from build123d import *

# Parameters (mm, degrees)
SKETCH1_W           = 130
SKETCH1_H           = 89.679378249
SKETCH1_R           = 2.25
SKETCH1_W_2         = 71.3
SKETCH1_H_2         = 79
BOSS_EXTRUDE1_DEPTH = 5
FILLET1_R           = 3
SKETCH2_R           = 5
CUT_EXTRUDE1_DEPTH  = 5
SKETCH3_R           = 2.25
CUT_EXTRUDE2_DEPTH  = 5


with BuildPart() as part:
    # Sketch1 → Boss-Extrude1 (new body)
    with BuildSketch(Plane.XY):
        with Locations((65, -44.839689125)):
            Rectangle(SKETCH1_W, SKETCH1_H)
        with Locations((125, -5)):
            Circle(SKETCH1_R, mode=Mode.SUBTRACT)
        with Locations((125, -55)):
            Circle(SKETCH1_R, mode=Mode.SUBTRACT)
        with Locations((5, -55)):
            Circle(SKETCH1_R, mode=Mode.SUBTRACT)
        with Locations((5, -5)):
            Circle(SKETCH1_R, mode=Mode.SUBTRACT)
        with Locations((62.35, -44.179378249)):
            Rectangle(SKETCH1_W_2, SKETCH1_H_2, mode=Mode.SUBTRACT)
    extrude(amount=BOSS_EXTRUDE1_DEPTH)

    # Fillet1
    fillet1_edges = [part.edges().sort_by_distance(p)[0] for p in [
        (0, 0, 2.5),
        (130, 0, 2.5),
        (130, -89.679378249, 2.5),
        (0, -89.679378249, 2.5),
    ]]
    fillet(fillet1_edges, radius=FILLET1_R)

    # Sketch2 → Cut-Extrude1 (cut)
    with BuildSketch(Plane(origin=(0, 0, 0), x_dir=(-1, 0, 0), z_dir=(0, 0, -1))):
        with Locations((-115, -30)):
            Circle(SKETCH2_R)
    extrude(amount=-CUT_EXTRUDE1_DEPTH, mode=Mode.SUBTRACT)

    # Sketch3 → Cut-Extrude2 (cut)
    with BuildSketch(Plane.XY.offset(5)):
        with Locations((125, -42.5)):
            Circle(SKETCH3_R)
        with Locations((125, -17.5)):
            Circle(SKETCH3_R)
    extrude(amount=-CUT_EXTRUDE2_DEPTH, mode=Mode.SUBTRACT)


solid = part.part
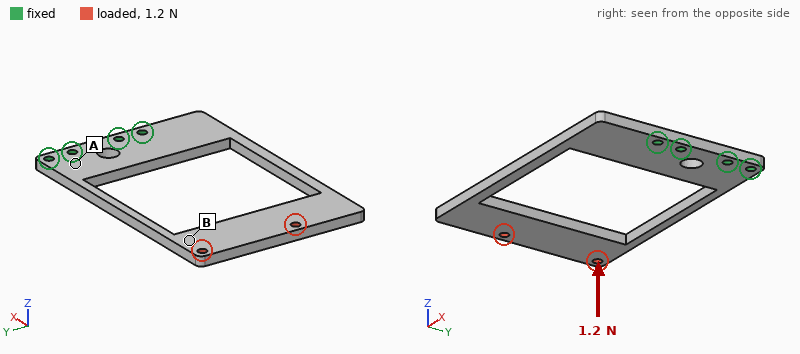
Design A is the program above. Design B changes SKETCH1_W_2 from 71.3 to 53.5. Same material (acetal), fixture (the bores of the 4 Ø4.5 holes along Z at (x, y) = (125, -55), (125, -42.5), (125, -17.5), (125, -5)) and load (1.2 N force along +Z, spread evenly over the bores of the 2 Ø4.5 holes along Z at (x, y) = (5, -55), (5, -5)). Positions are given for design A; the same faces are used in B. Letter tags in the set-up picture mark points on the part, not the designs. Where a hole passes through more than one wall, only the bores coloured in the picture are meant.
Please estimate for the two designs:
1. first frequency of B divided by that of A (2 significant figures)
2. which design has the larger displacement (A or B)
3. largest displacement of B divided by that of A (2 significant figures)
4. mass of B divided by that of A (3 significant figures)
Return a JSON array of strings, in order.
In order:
["1.1", "A", "0.79", "1.24"]
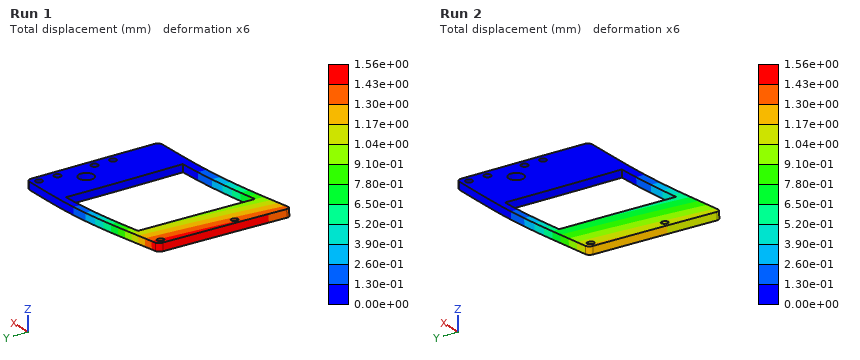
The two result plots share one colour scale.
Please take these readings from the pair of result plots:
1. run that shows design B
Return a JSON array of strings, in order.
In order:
["Run 2"]
